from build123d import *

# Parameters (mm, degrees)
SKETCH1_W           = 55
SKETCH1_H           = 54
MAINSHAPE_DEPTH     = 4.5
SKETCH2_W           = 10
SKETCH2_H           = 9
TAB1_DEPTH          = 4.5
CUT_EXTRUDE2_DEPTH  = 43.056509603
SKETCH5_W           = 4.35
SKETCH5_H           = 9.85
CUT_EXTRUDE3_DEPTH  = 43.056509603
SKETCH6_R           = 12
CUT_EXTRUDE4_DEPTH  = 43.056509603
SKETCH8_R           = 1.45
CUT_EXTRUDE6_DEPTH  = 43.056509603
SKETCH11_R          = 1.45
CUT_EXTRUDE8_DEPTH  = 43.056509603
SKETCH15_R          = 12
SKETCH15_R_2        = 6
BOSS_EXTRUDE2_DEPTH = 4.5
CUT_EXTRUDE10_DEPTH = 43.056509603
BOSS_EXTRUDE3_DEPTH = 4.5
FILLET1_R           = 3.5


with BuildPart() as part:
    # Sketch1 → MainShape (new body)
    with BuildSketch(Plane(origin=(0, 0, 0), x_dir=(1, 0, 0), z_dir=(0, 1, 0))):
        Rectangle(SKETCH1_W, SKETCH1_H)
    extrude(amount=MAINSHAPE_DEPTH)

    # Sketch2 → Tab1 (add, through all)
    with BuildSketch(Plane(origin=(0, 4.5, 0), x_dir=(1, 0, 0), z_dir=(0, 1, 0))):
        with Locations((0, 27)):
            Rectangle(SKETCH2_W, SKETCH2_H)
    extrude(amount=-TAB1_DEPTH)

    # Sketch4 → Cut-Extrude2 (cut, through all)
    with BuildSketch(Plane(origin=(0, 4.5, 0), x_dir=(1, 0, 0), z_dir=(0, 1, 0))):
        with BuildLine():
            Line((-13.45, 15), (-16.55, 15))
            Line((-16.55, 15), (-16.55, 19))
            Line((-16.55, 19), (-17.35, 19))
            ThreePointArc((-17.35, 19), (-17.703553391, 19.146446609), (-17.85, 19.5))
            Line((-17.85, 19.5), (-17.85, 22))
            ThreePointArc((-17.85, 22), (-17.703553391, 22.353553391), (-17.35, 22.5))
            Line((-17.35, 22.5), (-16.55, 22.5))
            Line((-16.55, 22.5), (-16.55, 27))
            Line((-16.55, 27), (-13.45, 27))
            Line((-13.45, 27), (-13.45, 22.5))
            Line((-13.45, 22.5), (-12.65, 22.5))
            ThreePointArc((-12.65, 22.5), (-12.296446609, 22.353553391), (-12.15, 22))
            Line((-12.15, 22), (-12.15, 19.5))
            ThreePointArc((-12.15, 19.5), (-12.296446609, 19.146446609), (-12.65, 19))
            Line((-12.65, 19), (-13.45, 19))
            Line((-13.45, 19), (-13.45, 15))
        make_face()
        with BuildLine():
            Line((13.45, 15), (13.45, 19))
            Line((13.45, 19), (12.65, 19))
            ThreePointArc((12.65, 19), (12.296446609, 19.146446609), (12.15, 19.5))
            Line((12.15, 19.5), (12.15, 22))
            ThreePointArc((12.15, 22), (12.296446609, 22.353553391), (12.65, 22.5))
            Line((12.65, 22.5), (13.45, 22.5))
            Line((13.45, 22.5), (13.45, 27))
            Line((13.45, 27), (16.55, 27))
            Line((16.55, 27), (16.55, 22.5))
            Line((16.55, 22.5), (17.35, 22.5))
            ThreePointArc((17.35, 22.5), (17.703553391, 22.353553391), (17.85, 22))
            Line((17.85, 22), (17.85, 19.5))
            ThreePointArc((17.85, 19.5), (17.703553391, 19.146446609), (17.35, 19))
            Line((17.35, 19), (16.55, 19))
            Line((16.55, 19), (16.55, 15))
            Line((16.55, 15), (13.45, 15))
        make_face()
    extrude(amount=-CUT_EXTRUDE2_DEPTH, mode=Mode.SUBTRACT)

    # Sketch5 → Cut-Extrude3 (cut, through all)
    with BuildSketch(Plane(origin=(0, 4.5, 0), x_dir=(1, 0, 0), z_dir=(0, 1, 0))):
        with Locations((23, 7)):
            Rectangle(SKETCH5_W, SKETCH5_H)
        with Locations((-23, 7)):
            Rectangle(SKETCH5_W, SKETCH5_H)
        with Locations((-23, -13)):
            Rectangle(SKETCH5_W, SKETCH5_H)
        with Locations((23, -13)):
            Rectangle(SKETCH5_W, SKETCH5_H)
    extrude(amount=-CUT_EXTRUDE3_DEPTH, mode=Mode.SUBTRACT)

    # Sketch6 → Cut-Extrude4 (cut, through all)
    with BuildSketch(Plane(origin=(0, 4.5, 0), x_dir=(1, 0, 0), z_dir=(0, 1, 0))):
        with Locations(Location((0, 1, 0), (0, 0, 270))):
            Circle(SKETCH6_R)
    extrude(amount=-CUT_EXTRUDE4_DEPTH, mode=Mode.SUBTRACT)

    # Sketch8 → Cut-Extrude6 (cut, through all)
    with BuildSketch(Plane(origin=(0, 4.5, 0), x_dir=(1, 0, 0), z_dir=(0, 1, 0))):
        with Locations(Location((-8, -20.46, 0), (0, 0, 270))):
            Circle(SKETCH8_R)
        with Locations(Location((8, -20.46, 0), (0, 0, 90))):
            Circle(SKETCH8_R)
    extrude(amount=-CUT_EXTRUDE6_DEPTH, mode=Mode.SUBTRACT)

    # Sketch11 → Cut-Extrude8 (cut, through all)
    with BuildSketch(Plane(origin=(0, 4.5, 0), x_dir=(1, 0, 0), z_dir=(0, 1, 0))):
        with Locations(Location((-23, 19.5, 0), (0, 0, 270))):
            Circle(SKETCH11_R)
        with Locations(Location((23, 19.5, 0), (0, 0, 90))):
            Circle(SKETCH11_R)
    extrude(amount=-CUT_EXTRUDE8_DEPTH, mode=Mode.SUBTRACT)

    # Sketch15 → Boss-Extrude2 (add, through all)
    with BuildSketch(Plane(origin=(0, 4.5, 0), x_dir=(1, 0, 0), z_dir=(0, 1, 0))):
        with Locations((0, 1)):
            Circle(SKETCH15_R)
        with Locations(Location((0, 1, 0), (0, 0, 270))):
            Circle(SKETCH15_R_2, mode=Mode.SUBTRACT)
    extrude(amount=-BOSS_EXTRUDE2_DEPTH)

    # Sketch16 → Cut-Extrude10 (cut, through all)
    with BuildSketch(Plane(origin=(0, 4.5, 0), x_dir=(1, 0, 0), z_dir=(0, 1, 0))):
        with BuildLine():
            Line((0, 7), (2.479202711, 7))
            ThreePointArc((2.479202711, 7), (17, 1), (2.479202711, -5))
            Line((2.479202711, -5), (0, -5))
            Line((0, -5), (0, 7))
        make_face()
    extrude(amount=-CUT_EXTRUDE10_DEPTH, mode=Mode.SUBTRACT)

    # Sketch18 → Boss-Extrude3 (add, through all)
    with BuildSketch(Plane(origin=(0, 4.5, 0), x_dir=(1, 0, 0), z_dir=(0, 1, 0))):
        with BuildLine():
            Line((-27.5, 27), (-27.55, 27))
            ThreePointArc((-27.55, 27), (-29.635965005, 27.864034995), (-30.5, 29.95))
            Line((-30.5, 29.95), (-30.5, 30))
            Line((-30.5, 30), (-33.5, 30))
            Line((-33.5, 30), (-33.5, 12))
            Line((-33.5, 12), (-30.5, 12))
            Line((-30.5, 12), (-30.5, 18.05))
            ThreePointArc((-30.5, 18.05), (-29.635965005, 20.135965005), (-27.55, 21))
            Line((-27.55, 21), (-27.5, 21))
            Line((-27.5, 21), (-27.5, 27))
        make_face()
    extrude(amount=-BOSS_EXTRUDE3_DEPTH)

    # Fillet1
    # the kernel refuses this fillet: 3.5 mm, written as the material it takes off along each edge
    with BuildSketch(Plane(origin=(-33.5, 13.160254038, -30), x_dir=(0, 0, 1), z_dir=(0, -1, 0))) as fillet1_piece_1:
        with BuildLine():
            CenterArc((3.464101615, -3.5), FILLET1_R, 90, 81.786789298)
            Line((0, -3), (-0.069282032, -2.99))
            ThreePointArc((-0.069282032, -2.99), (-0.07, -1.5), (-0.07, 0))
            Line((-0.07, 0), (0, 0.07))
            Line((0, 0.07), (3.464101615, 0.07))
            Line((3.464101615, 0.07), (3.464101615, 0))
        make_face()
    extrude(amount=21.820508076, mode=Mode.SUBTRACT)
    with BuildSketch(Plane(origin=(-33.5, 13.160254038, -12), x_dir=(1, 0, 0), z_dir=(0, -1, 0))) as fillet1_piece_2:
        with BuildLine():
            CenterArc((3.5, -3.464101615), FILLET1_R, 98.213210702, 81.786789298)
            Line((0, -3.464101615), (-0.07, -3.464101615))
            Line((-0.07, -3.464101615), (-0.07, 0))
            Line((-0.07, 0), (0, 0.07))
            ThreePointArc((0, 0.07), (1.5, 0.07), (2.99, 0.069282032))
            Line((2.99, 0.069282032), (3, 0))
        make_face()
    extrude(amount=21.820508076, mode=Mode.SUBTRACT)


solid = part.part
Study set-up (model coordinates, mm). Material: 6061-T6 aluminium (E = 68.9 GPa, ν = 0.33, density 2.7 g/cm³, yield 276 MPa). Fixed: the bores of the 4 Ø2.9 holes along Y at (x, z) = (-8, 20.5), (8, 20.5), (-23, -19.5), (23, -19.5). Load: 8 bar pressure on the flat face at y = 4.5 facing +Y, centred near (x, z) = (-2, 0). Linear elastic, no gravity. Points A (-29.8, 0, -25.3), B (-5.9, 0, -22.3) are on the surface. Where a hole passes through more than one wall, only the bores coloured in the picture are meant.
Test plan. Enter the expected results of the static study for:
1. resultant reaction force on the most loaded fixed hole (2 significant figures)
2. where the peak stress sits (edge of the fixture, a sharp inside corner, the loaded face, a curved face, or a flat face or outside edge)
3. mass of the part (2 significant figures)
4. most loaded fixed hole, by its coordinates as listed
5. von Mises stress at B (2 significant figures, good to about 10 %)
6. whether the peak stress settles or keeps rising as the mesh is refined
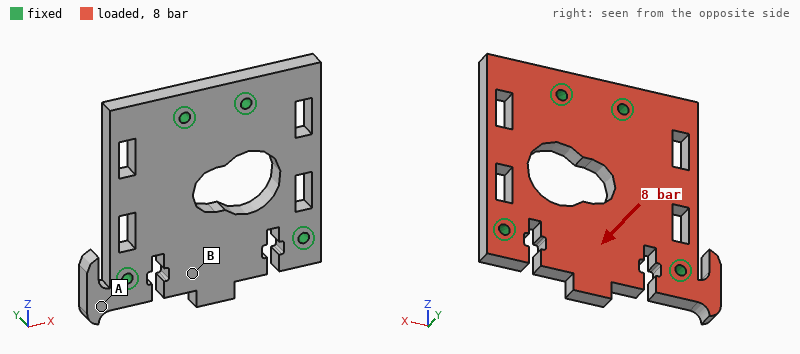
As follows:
590 N
edge of the fixture
30 g
(-23, -19.5)
22 MPa
keeps rising
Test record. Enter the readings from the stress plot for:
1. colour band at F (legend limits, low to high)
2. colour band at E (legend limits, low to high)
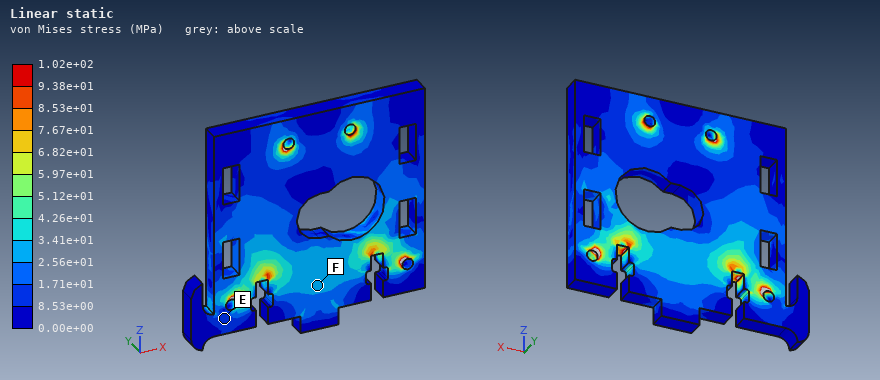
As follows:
2.56e+01 to 3.41e+01 MPa
8.53e+00 to 1.71e+01 MPa
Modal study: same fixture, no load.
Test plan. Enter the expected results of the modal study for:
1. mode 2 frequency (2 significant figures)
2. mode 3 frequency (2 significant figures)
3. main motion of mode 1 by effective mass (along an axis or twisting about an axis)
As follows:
9100 Hz
9200 Hz
along Y
